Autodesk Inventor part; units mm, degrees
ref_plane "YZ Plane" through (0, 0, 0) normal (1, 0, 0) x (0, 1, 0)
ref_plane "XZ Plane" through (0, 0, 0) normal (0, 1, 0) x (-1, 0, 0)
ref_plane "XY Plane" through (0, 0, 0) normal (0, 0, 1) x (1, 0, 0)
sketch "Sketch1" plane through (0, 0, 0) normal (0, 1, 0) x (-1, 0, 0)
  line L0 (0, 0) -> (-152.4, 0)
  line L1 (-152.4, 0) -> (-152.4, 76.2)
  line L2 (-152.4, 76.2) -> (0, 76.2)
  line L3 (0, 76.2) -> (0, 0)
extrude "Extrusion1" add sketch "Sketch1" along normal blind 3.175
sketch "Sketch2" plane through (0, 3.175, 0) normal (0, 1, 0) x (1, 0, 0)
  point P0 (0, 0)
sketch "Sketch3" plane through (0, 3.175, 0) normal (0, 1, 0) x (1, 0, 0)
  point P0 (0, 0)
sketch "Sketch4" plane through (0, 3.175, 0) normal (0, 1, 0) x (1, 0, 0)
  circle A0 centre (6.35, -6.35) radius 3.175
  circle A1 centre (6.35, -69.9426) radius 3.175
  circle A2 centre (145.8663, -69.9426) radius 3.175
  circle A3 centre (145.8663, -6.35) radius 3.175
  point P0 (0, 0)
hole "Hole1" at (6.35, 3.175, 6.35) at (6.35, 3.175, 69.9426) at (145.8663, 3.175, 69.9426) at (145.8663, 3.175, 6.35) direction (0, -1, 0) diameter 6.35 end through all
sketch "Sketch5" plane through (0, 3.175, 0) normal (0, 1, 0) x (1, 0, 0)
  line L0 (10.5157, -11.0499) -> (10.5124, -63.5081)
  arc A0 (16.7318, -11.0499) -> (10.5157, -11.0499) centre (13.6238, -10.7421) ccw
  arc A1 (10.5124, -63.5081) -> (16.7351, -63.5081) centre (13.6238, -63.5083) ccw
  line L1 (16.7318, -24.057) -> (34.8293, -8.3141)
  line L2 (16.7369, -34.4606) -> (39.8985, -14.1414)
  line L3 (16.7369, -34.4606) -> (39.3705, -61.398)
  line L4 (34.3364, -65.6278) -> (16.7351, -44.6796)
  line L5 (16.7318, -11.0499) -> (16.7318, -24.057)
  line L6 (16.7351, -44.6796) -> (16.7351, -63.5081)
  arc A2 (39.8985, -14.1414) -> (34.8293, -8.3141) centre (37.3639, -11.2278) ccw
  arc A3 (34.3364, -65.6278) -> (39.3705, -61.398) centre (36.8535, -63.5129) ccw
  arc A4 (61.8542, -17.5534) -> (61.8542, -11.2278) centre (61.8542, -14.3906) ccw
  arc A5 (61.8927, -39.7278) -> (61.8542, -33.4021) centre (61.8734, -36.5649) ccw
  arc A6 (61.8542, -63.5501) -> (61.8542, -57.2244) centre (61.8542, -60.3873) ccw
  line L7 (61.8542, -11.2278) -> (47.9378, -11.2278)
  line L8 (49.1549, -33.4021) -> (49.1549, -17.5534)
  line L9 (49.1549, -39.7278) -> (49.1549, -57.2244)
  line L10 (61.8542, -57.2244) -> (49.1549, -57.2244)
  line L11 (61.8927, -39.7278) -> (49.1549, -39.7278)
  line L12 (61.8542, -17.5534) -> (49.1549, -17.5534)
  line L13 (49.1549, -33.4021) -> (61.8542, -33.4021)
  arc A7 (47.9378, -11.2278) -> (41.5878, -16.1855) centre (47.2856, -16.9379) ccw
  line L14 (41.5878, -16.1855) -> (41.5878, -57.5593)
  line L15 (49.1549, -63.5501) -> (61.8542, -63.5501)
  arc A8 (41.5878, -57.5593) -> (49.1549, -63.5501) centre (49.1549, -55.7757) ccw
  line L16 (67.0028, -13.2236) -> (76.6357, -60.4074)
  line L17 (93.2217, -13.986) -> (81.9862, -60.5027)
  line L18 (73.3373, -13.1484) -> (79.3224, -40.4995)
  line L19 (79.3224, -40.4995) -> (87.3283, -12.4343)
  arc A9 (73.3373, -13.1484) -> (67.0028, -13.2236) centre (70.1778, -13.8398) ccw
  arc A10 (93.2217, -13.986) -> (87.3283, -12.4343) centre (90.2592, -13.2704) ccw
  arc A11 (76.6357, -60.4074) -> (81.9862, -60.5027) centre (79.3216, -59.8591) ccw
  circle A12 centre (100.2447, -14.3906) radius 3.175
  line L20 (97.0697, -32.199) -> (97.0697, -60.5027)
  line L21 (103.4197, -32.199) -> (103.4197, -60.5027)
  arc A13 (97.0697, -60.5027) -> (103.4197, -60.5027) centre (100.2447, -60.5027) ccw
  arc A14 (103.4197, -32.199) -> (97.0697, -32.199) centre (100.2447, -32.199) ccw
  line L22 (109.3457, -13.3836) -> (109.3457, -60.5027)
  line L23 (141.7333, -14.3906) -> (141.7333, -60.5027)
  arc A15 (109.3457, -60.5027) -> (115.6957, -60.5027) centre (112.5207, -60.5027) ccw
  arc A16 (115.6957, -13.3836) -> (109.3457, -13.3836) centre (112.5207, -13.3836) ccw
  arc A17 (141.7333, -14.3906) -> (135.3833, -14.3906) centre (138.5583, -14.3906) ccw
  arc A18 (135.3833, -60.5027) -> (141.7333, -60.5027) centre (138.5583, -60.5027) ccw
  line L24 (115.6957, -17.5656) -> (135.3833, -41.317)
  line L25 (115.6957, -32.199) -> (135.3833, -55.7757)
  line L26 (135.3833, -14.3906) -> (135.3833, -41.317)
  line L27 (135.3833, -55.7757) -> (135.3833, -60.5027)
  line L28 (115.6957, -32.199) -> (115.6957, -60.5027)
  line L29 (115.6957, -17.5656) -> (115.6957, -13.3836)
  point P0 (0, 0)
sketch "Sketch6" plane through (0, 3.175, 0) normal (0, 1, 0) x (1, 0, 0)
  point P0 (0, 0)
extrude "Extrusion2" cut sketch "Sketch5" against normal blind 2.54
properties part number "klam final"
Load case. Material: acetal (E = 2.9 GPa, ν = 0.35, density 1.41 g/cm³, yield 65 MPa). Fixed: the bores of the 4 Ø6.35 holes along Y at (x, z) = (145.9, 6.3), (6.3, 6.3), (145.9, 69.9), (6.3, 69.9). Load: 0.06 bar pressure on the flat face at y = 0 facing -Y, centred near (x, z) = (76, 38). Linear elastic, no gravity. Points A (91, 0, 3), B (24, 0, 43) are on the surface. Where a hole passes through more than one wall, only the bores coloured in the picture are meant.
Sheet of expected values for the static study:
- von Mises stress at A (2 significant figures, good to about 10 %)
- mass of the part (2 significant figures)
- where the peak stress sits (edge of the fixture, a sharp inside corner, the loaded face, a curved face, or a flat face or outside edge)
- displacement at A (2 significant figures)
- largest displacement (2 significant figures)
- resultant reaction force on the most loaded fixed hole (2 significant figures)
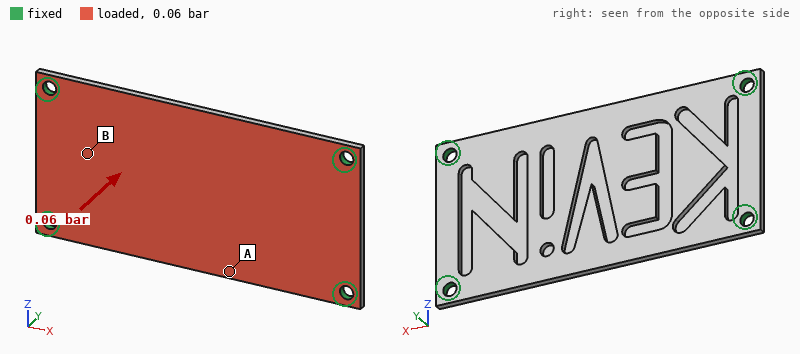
4.6 MPa
40 g
a curved face
1.3 mm
1.6 mm
29 N
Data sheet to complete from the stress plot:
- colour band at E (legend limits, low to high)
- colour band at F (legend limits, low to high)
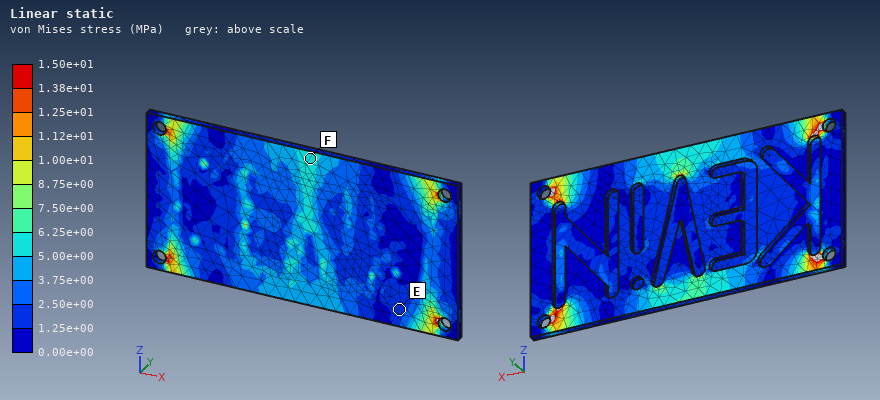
1.25e+00 to 2.50e+00 MPa
5.00e+00 to 6.25e+00 MPa
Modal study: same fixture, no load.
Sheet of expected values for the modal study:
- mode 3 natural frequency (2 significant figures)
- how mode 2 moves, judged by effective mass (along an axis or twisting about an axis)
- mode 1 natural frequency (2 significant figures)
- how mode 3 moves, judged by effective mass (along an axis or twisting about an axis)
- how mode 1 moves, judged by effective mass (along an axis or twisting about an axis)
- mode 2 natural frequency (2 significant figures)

500 Hz
twisting about X
200 Hz
twisting about Z
along Y
330 Hz
